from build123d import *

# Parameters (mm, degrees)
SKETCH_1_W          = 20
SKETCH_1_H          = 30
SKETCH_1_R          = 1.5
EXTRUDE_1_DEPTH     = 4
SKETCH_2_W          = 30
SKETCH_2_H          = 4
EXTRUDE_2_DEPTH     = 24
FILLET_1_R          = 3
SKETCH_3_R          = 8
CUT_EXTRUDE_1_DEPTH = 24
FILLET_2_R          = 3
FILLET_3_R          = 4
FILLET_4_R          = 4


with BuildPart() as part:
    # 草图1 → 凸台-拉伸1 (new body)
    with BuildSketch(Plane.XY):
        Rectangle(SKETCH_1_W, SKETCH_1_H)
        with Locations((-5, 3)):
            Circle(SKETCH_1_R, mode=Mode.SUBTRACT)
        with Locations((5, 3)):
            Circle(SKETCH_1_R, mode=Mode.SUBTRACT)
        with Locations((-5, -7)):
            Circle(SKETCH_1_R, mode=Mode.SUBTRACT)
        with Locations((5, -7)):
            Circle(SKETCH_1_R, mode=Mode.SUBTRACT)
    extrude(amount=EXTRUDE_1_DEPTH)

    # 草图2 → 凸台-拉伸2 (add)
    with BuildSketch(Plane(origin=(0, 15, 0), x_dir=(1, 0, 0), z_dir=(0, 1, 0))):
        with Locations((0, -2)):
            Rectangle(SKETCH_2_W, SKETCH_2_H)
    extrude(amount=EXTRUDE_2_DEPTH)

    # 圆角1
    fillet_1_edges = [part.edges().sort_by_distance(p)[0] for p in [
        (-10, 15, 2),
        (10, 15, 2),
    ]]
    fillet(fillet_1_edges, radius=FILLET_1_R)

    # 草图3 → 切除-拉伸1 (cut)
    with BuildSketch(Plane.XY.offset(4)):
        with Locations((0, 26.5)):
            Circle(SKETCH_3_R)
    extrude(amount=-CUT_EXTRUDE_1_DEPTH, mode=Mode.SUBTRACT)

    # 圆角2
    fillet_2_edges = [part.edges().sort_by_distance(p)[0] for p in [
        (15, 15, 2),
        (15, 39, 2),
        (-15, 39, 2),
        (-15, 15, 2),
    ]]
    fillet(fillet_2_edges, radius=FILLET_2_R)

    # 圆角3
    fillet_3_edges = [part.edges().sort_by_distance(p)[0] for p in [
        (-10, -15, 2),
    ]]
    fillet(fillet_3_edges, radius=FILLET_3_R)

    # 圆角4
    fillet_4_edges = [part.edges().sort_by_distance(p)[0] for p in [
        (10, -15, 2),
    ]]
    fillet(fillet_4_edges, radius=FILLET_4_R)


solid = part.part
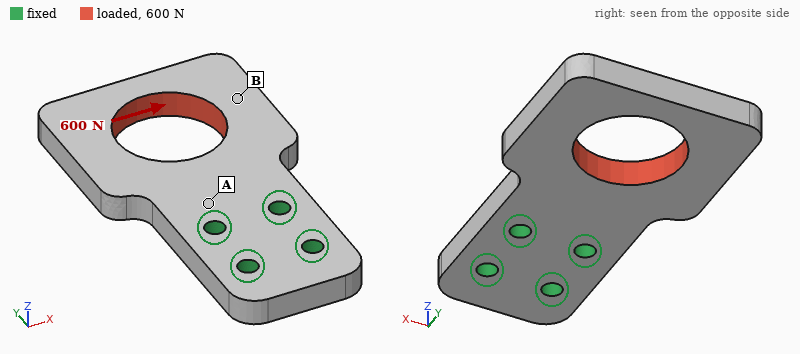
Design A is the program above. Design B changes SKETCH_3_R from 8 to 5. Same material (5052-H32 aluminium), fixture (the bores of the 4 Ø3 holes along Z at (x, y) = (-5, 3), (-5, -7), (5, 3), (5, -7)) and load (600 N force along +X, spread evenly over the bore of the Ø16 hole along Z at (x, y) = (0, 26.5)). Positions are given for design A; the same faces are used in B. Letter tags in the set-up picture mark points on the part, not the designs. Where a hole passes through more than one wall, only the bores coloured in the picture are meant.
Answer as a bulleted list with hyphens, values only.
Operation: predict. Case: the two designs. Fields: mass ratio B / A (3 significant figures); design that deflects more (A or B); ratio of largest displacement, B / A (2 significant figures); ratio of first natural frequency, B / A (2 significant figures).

- 1.11
- A
- 0.72
- 0.96
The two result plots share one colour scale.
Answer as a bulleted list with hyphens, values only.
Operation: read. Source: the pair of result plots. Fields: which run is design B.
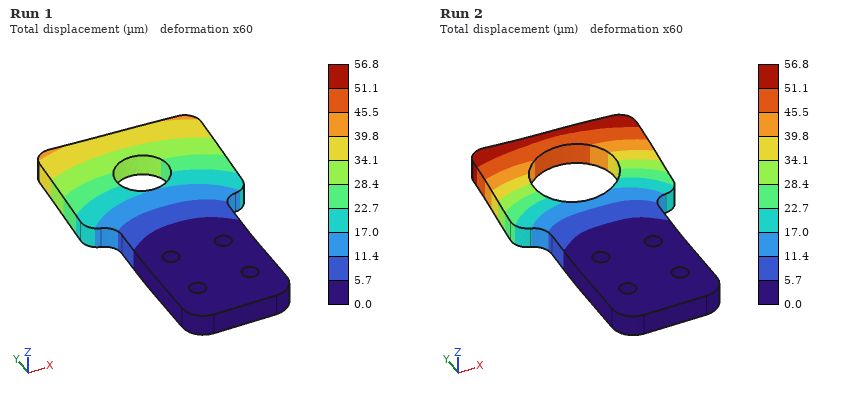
- Run 1
